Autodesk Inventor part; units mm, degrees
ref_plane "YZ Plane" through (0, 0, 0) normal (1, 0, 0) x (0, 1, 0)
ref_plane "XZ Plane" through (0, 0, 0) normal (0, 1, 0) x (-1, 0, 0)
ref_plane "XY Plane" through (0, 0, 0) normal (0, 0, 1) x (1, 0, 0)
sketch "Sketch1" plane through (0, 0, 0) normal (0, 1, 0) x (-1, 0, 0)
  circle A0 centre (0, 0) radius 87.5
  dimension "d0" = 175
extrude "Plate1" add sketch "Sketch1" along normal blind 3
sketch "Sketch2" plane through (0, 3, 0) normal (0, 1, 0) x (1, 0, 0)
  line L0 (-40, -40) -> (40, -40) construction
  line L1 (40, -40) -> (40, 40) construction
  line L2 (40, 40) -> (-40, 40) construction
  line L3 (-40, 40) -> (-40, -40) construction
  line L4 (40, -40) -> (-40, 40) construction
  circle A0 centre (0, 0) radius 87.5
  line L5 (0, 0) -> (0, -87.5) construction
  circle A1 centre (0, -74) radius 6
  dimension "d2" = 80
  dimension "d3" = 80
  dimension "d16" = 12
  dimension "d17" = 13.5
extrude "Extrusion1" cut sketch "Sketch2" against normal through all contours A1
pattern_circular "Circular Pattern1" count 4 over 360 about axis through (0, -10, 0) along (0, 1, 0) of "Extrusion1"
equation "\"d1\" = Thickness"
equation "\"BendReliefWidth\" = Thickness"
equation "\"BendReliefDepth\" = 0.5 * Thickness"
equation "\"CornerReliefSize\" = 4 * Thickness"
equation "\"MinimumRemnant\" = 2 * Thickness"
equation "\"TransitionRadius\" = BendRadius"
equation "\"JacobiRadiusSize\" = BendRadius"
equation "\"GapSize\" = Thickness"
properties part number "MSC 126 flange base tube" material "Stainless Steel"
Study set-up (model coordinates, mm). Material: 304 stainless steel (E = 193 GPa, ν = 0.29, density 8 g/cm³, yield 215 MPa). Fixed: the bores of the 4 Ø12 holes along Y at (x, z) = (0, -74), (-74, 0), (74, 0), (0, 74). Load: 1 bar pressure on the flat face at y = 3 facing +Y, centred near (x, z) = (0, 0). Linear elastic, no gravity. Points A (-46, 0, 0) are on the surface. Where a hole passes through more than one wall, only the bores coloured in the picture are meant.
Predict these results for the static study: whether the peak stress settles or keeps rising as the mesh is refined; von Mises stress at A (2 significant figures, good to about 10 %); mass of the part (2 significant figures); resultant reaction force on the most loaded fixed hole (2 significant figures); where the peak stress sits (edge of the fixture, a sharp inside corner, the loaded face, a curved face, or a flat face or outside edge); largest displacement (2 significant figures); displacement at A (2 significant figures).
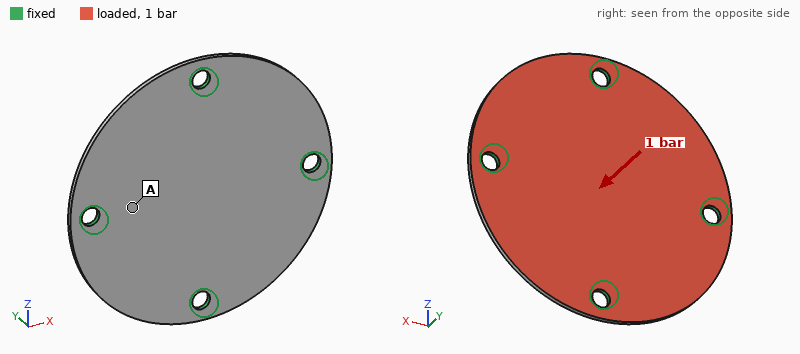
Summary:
keeps rising
18 MPa
570 g
590 N
edge of the fixture
0.12 mm
0.053 mm
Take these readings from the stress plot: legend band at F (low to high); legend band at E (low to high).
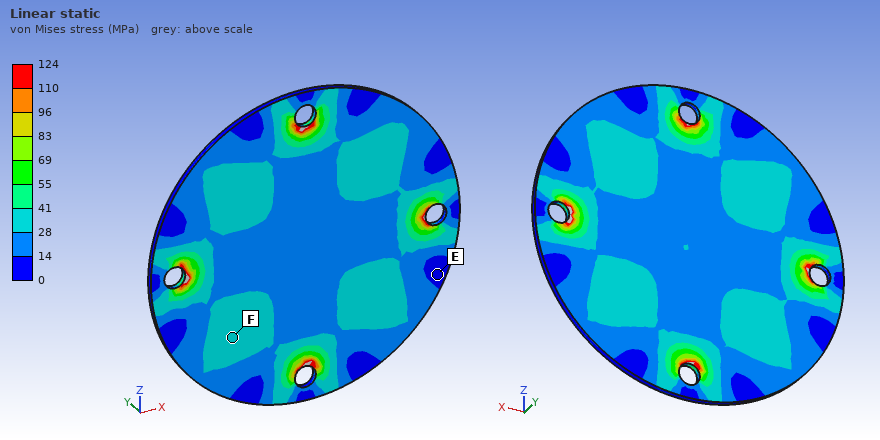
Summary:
28 to 41 MPa
0 to 14 MPa
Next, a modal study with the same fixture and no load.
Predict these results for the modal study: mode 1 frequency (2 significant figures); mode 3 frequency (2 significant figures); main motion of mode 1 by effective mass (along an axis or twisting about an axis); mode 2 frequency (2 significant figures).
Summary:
1100 Hz
1300 Hz
along Y
1300 Hz
